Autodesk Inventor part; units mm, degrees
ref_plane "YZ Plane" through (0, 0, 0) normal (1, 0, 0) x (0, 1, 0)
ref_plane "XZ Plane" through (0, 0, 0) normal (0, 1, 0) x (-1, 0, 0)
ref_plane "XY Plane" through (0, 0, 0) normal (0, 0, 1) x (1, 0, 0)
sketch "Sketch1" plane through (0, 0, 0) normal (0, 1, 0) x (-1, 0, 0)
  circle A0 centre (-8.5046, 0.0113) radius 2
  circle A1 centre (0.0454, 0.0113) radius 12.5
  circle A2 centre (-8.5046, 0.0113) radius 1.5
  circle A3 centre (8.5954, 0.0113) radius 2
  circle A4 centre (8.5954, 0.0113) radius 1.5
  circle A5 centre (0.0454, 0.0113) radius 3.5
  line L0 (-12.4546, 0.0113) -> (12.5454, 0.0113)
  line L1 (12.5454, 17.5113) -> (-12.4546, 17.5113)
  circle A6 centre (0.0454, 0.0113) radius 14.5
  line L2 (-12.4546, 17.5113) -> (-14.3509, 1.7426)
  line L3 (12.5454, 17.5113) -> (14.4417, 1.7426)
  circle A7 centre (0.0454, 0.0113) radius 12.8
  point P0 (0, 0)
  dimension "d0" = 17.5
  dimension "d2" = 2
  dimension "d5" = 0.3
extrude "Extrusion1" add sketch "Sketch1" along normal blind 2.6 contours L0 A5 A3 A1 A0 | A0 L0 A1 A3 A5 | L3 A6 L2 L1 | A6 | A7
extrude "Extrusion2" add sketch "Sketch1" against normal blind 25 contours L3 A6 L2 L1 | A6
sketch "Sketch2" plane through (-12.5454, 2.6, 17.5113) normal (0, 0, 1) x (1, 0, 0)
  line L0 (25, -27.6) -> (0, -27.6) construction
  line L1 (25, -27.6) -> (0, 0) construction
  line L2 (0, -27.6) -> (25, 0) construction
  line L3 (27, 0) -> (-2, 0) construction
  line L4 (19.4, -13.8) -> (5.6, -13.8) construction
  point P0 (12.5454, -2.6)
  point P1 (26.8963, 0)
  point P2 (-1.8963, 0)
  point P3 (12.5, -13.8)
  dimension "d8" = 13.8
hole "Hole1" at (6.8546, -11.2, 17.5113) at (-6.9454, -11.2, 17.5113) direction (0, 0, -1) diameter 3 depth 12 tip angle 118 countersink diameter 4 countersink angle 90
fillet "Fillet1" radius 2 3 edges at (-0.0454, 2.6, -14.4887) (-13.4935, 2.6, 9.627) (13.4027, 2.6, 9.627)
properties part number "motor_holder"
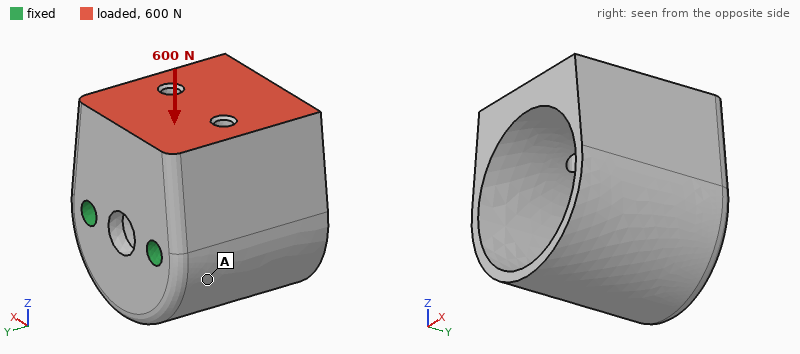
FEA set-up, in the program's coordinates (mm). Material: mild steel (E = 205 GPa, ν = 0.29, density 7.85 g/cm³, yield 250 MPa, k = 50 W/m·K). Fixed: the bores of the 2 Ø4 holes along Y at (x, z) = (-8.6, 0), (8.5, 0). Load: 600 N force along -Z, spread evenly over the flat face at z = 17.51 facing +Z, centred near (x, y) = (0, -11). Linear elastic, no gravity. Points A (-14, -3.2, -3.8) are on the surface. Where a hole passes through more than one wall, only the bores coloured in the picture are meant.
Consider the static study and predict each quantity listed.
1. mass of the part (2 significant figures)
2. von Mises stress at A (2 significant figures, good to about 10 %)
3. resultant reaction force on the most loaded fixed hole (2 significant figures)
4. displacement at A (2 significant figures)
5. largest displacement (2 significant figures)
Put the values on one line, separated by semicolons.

71 g; 22 MPa; 300 N; 6.9 µm; 38 µm
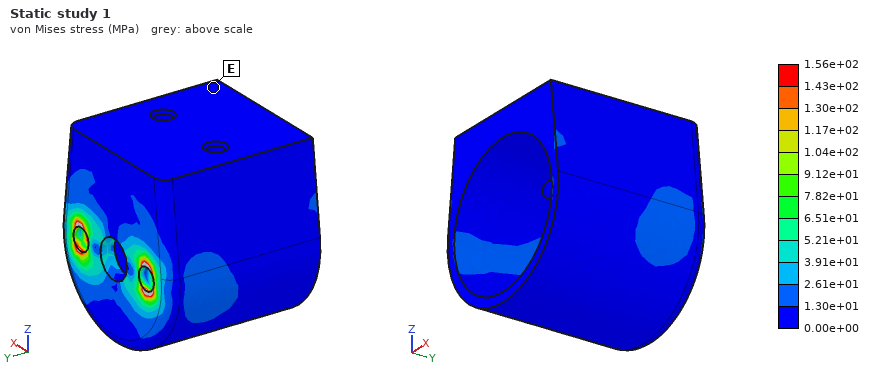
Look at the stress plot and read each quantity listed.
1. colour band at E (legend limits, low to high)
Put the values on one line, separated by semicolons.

0.00e+00 to 1.30e+01 MPa
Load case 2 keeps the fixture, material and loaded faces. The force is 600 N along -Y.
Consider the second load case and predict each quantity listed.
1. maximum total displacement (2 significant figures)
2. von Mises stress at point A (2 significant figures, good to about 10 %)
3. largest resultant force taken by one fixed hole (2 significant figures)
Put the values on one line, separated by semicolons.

50 µm; 25 MPa; 300 N
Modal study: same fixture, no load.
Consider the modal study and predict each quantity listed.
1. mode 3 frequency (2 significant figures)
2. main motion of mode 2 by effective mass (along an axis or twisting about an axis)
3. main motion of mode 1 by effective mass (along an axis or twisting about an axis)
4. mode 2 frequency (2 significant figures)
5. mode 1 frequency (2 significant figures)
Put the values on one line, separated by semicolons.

9700 Hz; along X; along Z; 6300 Hz; 2700 Hz
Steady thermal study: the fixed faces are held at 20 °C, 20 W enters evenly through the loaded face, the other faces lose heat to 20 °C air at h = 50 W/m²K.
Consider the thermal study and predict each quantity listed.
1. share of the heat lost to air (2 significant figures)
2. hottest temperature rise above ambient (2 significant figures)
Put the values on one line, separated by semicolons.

32 %; 45 K
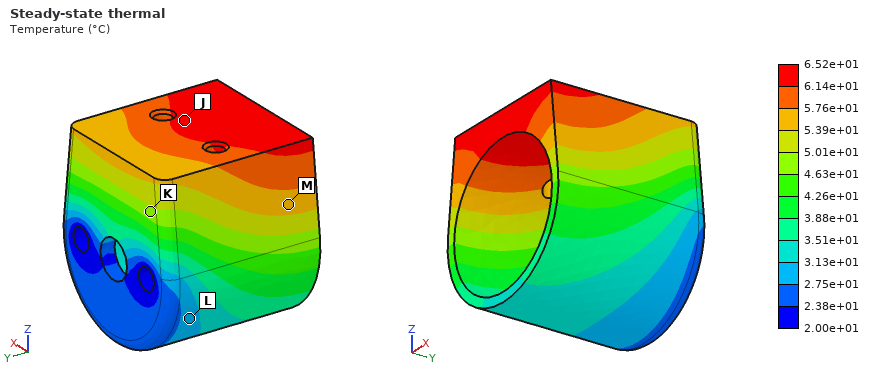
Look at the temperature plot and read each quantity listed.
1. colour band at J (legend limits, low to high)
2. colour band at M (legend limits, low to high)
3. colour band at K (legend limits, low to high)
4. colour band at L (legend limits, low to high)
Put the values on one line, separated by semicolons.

6.14e+01 to 6.52e+01 °C; 5.39e+01 to 5.76e+01 °C; 4.63e+01 to 5.01e+01 °C; 2.75e+01 to 3.13e+01 °C
